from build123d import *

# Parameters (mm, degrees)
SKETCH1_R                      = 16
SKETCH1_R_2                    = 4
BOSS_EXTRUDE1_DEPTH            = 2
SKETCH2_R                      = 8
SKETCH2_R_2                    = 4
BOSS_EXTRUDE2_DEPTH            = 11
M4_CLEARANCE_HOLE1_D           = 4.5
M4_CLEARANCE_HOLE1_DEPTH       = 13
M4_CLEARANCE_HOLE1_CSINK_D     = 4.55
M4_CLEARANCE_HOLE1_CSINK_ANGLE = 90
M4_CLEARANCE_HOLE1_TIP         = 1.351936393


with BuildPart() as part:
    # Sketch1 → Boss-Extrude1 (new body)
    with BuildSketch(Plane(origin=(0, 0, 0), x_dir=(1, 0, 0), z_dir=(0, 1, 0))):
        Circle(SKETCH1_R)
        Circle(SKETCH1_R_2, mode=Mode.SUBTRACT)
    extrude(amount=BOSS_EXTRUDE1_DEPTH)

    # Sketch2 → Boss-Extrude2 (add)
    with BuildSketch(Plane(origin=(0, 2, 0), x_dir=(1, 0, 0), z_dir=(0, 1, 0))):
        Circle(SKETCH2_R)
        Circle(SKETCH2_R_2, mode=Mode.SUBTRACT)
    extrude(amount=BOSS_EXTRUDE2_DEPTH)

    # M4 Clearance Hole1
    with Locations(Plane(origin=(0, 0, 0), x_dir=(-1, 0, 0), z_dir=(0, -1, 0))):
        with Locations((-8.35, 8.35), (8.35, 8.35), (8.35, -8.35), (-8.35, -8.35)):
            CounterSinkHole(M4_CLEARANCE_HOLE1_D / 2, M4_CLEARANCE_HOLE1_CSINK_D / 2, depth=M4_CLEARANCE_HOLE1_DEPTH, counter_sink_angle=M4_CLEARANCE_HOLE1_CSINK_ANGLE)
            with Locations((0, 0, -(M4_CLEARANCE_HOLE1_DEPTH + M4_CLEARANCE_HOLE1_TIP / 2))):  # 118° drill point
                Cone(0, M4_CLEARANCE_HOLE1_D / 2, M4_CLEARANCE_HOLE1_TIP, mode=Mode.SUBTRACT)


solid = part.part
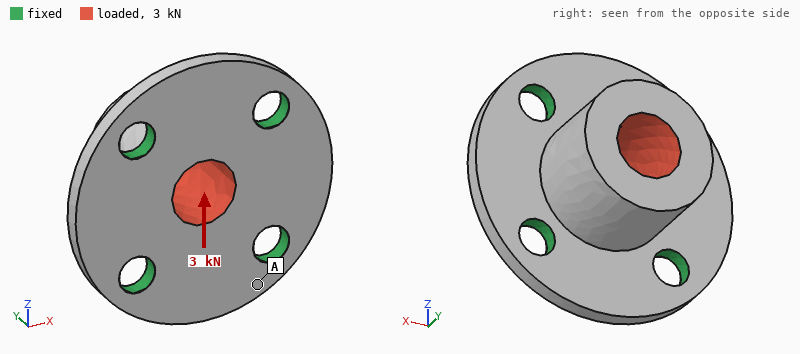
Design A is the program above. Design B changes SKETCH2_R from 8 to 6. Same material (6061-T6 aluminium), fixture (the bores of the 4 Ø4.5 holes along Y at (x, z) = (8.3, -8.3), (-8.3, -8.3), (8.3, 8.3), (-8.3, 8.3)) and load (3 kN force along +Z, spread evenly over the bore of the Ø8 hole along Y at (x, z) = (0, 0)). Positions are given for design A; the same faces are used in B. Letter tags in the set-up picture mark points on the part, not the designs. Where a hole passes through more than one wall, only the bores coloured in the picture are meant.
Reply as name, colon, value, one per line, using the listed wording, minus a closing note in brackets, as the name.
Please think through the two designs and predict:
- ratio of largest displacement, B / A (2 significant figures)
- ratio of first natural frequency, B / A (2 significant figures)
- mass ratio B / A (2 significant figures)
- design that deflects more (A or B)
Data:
ratio of largest displacement, B / A: 3.1
ratio of first natural frequency, B / A: 0.88
mass ratio B / A: 0.68
design that deflects more: B
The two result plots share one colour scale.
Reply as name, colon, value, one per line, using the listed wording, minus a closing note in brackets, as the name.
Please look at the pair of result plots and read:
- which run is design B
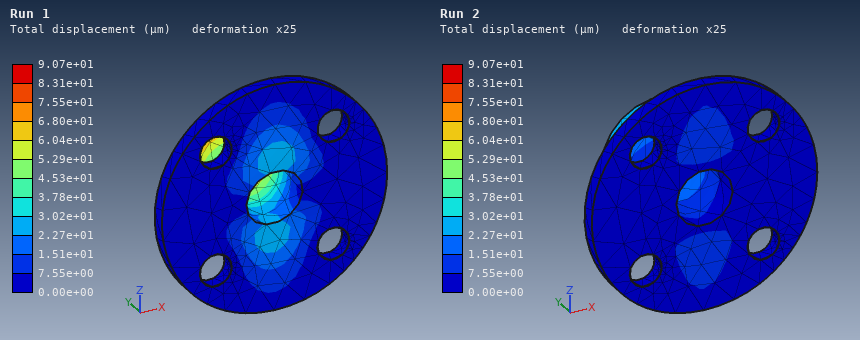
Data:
which run is design B: Run 1
